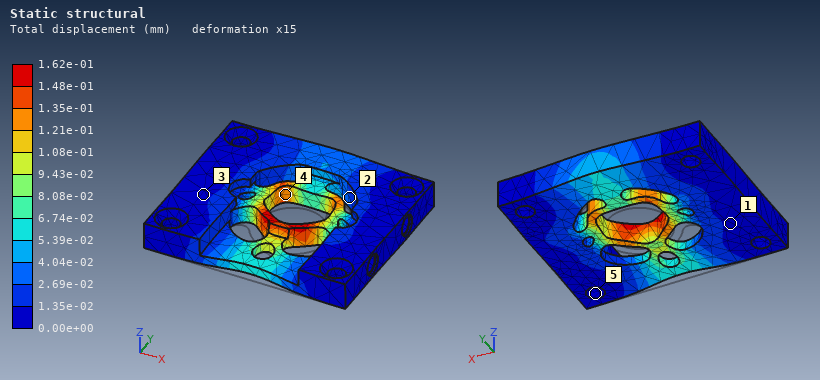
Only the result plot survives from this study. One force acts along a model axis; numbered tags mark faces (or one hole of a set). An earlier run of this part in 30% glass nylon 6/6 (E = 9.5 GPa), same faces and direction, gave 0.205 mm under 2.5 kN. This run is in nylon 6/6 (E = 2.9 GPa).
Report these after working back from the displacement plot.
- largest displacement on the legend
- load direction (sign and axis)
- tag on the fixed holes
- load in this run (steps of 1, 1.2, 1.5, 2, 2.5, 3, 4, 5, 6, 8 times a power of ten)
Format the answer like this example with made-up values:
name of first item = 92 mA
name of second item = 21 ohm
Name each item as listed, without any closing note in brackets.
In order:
largest displacement on the legend = 1.62e-01 mm
load direction = +Y
tag on the fixed holes = 5
load in this run = 600 N
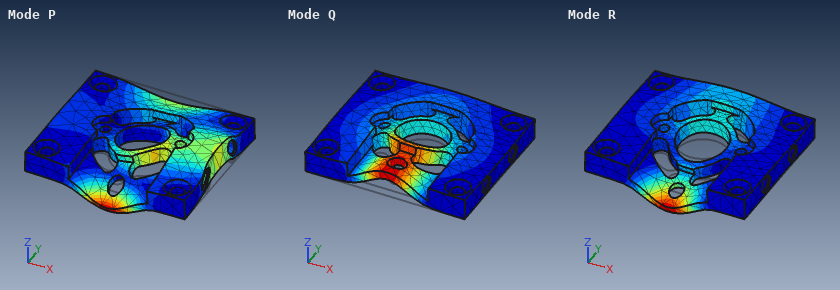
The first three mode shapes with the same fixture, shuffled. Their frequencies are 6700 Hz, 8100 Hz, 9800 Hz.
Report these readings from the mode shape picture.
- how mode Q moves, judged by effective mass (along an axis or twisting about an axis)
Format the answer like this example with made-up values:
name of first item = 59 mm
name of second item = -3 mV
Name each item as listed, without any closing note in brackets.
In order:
how mode Q moves, judged by effective mass = along Z
